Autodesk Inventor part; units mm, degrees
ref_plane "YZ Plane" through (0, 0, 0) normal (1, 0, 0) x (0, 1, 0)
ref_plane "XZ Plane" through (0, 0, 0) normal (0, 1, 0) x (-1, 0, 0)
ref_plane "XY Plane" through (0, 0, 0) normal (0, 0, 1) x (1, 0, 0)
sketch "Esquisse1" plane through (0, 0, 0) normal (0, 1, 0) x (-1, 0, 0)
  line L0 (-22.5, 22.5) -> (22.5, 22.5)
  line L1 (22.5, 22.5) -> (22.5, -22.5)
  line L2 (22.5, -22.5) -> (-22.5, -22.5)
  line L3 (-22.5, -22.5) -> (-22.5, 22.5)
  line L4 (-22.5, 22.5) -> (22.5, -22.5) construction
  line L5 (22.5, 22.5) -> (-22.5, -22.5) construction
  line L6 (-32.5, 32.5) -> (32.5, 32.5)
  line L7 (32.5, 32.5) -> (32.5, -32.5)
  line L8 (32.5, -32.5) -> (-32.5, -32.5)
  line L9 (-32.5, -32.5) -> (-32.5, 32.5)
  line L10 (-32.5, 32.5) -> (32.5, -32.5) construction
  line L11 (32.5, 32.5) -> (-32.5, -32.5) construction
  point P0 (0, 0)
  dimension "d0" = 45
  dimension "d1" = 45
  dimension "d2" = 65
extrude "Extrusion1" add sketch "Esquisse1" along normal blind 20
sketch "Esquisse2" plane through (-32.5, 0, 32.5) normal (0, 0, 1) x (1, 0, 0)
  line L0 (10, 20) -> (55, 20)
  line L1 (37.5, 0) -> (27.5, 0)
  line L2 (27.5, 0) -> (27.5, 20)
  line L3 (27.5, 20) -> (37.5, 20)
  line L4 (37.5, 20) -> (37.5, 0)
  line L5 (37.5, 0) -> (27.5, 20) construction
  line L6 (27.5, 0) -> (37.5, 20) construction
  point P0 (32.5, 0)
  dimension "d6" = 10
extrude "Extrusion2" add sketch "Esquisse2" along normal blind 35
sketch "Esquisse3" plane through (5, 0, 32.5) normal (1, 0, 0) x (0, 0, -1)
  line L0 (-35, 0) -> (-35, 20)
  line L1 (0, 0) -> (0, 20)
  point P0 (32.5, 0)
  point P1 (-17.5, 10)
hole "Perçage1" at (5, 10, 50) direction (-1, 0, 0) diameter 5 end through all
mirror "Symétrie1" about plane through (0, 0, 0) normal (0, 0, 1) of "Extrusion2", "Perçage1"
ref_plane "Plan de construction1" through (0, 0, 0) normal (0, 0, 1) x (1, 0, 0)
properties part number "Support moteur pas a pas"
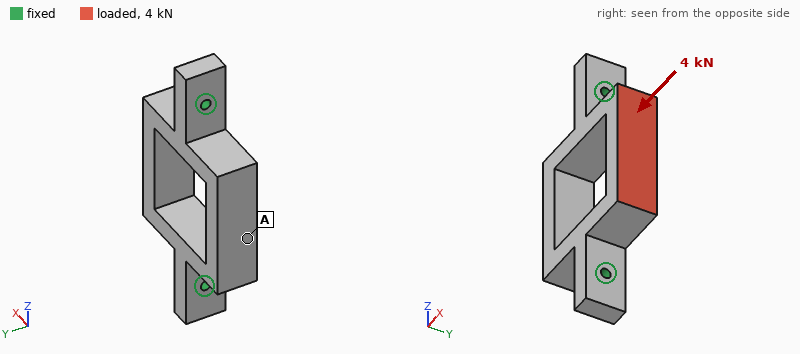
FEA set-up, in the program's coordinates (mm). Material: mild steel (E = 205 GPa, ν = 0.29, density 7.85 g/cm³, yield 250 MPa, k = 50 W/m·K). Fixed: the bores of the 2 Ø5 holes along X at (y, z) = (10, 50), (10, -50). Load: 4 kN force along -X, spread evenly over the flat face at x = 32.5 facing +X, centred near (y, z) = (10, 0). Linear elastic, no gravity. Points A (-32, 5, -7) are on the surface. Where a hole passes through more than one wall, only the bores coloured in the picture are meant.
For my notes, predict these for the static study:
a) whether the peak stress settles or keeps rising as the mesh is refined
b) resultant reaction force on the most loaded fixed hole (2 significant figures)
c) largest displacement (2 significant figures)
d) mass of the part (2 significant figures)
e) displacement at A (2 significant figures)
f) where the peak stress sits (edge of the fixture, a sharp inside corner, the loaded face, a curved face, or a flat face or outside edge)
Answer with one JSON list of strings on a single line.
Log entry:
["keeps rising", "2.1 kN", "16 µm", "450 g", "6.9 µm", "edge of the fixture"]
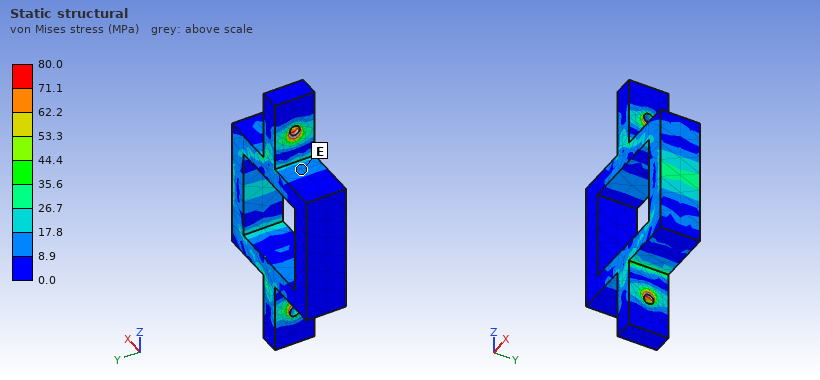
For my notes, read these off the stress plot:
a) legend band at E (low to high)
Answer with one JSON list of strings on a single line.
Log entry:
["8.9 to 17.8 MPa"]
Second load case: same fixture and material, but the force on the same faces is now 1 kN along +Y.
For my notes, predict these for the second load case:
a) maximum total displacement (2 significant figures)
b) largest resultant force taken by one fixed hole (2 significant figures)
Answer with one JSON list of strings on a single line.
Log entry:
["37 µm", "500 N"]
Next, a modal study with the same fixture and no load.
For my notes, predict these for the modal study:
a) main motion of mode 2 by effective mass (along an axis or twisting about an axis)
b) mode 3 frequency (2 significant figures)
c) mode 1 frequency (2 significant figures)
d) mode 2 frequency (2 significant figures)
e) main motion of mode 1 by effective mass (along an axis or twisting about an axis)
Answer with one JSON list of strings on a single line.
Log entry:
["along Y", "5200 Hz", "2300 Hz", "3800 Hz", "twisting about Z"]
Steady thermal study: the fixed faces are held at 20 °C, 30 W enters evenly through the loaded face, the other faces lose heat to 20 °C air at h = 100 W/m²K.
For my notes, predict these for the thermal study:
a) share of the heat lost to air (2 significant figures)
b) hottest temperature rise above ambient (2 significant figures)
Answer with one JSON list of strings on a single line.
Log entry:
["66 %", "44 K"]
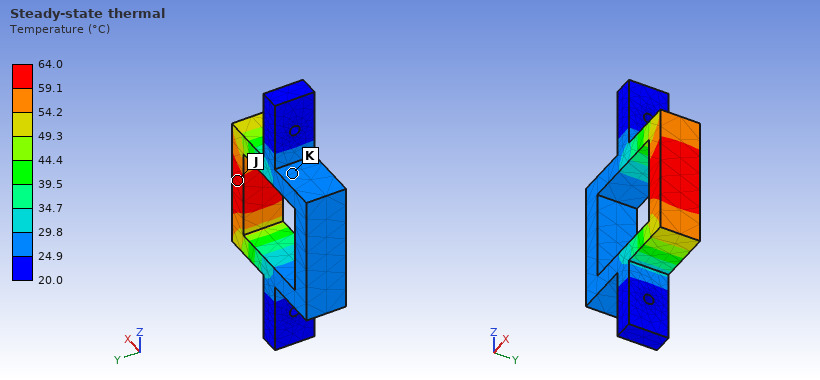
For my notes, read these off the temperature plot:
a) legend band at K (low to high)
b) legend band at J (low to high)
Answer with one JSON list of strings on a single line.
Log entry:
["24.9 to 29.8 °C", "59.1 to 64.0 °C"]
